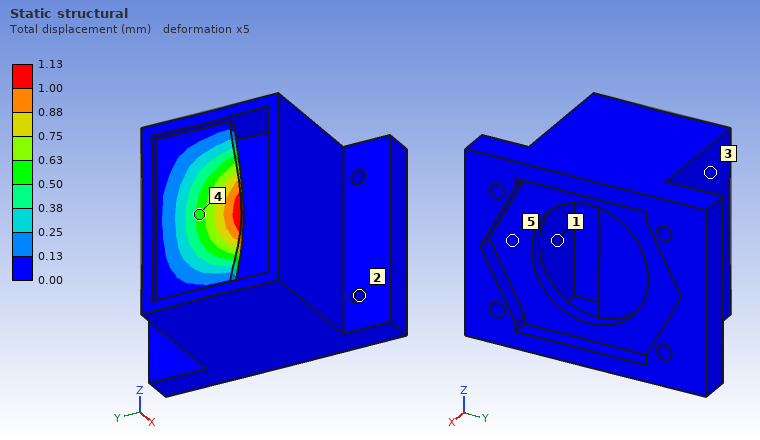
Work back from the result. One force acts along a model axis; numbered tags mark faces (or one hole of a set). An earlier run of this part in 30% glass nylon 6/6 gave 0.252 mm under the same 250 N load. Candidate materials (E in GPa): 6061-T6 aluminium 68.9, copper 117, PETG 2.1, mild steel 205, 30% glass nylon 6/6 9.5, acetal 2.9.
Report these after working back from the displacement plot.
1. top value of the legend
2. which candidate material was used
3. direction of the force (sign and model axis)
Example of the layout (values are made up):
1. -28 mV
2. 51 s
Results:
1. 1.13 mm
2. PETG
3. +X
